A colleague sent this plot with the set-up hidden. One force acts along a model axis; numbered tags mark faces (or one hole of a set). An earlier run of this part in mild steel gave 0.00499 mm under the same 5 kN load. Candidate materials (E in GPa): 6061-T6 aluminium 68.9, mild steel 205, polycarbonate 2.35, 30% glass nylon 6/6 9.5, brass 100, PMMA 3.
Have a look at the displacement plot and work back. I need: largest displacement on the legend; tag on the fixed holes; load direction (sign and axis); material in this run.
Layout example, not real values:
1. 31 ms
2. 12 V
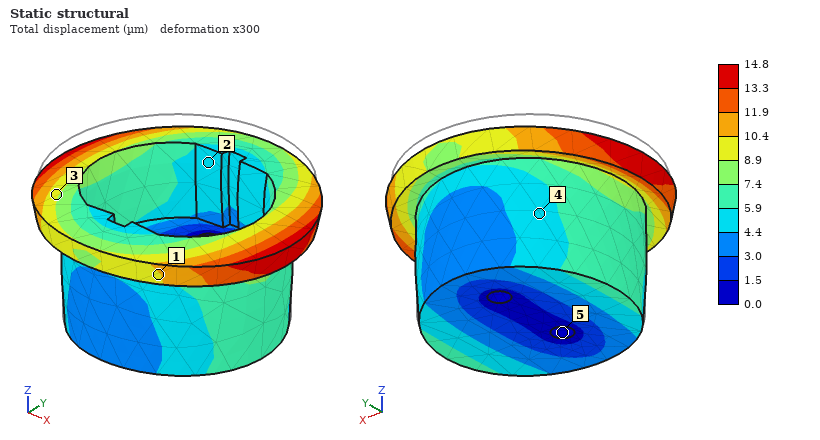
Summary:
1. 14.8 µm
2. 5
3. -Z
4. 6061-T6 aluminium
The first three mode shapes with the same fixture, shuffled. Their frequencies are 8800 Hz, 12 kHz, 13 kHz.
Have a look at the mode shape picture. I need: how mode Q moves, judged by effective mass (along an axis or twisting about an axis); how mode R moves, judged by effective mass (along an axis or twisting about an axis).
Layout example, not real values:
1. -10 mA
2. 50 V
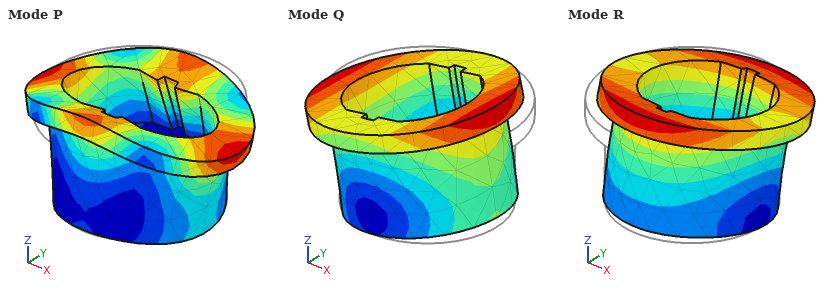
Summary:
1. along X
2. along Y
